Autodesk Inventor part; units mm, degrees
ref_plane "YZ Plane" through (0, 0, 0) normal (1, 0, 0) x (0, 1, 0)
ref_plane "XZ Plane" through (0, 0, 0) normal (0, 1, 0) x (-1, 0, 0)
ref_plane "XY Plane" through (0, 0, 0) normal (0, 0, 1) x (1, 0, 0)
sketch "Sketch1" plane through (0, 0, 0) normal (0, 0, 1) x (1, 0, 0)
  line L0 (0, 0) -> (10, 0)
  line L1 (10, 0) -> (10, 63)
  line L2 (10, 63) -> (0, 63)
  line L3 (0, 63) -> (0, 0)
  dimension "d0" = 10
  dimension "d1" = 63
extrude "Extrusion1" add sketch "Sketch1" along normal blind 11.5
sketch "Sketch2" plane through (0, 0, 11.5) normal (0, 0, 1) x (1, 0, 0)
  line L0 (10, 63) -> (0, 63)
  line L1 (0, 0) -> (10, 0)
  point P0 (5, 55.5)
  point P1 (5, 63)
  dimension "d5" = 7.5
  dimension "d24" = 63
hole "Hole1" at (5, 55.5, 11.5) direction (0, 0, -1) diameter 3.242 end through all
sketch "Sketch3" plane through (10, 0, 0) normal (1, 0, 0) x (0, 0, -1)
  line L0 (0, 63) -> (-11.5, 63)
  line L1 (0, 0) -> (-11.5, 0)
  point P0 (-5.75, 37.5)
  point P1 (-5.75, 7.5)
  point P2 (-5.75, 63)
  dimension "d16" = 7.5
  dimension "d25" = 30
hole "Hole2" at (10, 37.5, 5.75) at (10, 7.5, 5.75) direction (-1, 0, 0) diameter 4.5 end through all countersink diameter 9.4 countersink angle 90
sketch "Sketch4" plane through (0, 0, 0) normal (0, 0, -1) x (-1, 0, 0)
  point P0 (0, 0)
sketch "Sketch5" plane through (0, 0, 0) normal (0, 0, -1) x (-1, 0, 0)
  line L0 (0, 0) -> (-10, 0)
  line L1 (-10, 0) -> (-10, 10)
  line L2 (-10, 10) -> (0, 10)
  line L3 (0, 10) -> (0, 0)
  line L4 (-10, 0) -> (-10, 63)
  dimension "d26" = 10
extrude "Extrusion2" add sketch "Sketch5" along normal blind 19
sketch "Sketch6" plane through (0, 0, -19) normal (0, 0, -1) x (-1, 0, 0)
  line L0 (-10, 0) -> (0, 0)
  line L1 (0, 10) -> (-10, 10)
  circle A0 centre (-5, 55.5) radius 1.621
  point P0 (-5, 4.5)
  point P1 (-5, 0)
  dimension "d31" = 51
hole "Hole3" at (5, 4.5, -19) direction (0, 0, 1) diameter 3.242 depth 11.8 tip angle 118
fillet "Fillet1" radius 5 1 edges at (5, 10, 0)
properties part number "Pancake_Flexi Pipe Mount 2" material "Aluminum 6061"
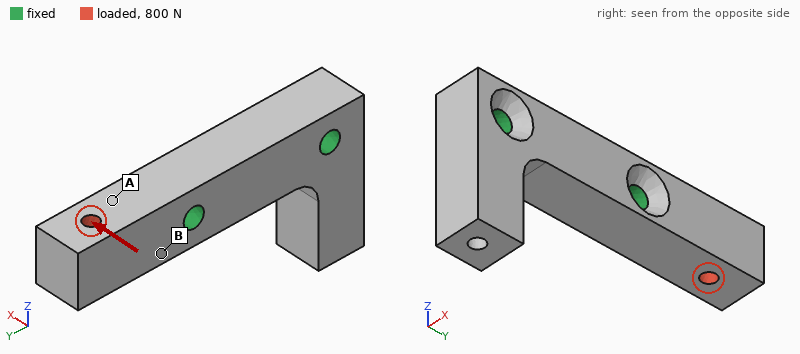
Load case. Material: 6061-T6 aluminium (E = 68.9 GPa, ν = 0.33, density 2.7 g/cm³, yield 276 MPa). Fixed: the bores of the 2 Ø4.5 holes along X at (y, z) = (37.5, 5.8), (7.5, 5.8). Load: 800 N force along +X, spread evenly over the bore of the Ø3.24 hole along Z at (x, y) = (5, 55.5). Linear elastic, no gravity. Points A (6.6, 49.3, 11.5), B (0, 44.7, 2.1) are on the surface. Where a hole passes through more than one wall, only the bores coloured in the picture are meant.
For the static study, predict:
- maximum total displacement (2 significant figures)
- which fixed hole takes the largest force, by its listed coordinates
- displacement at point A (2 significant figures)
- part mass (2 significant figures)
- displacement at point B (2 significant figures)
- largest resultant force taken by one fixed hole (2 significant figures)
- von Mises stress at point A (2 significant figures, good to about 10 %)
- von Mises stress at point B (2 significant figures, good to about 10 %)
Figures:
53 µm
(37.5, 5.8)
18 µm
23 g
11 µm
880 N
20 MPa
47 MPa
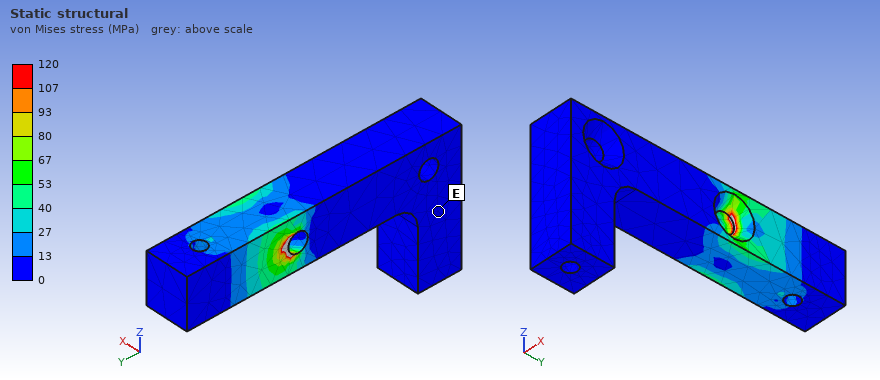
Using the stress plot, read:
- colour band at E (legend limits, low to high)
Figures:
0 to 13 MPa
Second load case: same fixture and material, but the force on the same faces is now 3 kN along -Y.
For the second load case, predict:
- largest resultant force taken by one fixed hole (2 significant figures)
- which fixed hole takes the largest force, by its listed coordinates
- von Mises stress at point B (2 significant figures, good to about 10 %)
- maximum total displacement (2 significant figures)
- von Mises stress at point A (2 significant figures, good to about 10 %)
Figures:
2.9 kN
(37.5, 5.8)
23 MPa
10 µm
27 MPa
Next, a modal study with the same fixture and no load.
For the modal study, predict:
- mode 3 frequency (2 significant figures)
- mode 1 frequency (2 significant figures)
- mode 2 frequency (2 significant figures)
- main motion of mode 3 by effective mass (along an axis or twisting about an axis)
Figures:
12 kHz
11 kHz
11 kHz
along X
